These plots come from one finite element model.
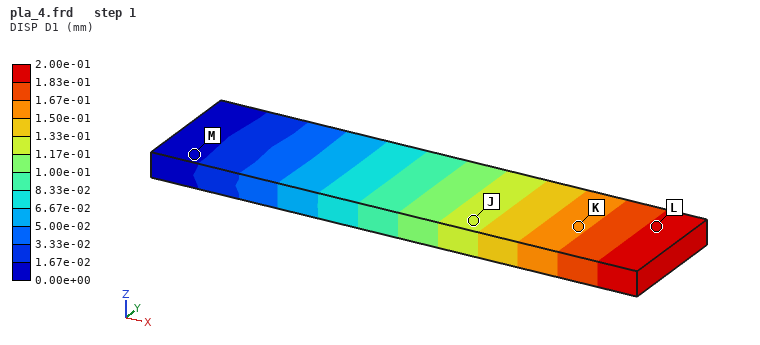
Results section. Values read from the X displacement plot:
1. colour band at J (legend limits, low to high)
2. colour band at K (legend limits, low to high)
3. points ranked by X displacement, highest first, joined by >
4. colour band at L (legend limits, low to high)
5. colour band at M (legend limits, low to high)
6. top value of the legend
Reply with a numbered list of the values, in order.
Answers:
1. 1.17e-01 to 1.33e-01 mm
2. 1.50e-01 to 1.67e-01 mm
3. L > K > J > M
4. 1.83e-01 to 2.00e-01 mm
5. 0.00e+00 to 1.67e-02 mm
6. 2.00e-01 mm
